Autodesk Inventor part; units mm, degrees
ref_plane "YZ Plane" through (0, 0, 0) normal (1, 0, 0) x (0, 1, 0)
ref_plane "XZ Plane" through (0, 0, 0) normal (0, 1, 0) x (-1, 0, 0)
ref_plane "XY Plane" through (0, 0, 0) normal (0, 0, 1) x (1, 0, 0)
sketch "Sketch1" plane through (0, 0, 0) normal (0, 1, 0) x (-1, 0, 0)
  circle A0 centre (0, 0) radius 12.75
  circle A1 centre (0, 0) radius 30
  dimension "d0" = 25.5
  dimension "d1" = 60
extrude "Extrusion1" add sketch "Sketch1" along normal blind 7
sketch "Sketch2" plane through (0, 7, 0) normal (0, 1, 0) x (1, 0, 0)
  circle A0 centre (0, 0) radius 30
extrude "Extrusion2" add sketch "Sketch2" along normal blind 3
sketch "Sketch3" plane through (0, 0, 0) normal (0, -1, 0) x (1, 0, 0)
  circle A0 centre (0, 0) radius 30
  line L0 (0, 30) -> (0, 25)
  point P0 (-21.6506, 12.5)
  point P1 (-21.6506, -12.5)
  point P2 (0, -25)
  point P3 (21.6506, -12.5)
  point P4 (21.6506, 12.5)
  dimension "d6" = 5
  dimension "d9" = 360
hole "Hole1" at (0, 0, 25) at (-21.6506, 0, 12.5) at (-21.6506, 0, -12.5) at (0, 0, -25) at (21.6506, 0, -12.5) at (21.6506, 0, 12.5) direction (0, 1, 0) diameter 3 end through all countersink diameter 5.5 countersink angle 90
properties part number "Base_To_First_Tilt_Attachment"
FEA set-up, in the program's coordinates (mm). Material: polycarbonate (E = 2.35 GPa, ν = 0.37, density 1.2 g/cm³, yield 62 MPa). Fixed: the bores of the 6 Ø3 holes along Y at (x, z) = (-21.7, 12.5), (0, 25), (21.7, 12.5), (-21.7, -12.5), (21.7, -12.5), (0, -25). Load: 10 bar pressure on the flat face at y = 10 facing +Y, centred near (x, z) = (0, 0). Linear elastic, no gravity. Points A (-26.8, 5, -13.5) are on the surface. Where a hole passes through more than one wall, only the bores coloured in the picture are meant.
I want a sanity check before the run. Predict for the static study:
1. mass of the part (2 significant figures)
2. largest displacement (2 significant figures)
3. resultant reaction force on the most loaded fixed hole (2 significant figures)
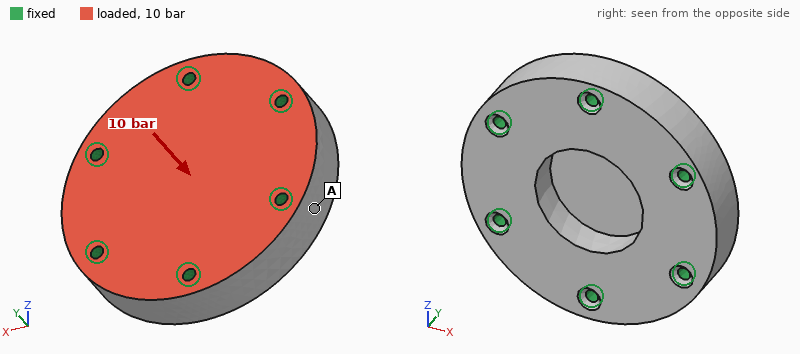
29 g
0.20 mm
470 N
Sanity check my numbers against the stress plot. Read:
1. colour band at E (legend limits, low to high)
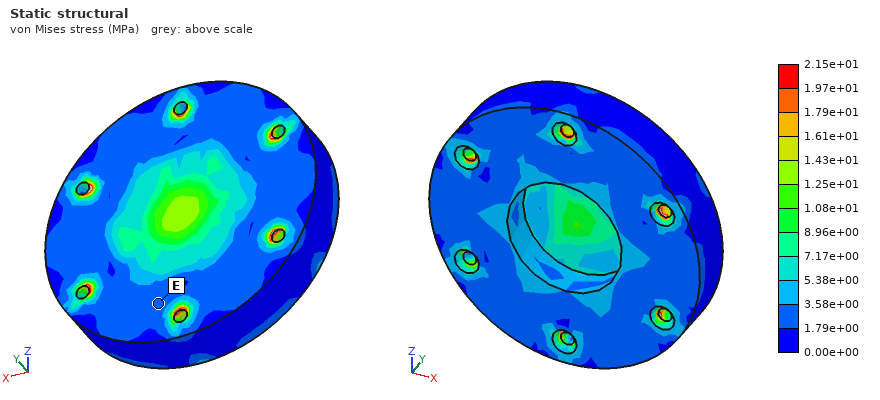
1.79e+00 to 3.58e+00 MPa
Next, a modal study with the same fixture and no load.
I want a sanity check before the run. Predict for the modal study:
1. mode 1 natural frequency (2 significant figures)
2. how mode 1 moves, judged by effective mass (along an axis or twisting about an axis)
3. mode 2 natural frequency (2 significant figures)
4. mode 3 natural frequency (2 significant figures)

6800 Hz
along Y
9700 Hz
9700 Hz
